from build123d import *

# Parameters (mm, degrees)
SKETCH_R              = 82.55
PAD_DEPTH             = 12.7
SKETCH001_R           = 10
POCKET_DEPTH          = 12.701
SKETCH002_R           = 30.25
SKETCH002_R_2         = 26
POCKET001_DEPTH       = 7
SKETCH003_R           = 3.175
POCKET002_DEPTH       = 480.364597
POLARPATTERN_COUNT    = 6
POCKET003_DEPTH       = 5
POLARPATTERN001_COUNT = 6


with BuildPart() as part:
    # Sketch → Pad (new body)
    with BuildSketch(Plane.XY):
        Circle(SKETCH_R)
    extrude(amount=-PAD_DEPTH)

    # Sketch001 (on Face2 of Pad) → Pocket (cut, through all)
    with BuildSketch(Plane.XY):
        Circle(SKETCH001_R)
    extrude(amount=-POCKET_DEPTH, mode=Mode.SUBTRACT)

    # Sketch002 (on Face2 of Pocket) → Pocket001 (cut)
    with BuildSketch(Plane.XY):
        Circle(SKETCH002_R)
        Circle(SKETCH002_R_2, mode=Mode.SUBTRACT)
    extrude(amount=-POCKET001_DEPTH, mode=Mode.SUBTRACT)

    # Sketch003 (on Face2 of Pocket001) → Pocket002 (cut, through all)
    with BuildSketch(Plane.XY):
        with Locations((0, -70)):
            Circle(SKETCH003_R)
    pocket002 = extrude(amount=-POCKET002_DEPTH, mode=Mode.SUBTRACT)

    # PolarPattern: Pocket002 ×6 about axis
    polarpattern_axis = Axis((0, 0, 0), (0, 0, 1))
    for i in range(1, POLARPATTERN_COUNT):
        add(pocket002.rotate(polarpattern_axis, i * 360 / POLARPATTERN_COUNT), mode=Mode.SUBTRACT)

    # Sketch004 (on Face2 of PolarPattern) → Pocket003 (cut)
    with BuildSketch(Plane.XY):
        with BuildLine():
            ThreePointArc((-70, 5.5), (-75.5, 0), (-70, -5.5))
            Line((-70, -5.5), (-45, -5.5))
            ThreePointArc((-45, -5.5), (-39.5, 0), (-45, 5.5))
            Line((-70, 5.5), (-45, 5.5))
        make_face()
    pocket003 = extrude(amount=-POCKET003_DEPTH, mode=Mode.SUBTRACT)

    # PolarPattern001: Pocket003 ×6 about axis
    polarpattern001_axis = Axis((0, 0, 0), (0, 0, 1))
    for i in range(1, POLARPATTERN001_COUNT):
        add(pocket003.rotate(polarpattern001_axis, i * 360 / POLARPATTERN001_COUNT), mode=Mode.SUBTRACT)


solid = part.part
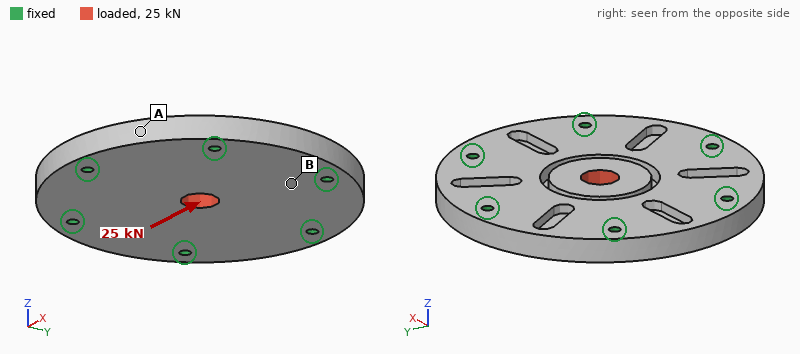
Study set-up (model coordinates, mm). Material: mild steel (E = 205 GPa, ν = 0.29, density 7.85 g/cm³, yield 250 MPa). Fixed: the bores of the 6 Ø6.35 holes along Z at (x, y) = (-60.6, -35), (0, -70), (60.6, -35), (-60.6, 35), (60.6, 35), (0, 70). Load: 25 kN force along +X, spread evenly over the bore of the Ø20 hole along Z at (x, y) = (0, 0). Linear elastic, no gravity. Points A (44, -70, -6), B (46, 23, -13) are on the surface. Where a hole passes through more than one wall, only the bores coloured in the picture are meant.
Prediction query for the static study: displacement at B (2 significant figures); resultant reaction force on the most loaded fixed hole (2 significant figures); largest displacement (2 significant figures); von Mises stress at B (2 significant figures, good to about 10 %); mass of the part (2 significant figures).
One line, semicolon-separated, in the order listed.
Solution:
3.0 µm; 5.4 kN; 12 µm; 24 MPa; 2.0 kg
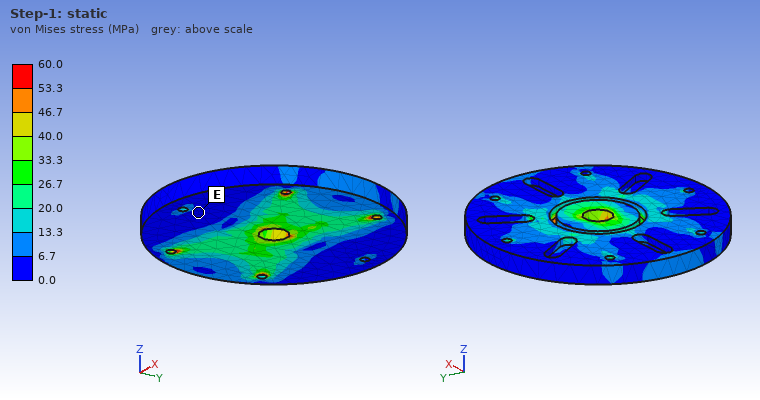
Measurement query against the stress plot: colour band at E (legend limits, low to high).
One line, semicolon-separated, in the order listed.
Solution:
0.0 to 6.7 MPa
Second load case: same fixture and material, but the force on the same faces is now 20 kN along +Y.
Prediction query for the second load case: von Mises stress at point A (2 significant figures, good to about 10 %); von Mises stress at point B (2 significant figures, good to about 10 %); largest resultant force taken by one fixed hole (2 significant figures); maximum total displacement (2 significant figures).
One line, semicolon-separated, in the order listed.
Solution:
6.0 MPa; 10 MPa; 4.9 kN; 9.9 µm
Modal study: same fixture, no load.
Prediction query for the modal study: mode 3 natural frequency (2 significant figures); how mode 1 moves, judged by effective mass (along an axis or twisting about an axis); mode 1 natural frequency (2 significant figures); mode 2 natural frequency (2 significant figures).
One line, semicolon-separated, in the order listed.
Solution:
7700 Hz; along Z; 4600 Hz; 7700 Hz
